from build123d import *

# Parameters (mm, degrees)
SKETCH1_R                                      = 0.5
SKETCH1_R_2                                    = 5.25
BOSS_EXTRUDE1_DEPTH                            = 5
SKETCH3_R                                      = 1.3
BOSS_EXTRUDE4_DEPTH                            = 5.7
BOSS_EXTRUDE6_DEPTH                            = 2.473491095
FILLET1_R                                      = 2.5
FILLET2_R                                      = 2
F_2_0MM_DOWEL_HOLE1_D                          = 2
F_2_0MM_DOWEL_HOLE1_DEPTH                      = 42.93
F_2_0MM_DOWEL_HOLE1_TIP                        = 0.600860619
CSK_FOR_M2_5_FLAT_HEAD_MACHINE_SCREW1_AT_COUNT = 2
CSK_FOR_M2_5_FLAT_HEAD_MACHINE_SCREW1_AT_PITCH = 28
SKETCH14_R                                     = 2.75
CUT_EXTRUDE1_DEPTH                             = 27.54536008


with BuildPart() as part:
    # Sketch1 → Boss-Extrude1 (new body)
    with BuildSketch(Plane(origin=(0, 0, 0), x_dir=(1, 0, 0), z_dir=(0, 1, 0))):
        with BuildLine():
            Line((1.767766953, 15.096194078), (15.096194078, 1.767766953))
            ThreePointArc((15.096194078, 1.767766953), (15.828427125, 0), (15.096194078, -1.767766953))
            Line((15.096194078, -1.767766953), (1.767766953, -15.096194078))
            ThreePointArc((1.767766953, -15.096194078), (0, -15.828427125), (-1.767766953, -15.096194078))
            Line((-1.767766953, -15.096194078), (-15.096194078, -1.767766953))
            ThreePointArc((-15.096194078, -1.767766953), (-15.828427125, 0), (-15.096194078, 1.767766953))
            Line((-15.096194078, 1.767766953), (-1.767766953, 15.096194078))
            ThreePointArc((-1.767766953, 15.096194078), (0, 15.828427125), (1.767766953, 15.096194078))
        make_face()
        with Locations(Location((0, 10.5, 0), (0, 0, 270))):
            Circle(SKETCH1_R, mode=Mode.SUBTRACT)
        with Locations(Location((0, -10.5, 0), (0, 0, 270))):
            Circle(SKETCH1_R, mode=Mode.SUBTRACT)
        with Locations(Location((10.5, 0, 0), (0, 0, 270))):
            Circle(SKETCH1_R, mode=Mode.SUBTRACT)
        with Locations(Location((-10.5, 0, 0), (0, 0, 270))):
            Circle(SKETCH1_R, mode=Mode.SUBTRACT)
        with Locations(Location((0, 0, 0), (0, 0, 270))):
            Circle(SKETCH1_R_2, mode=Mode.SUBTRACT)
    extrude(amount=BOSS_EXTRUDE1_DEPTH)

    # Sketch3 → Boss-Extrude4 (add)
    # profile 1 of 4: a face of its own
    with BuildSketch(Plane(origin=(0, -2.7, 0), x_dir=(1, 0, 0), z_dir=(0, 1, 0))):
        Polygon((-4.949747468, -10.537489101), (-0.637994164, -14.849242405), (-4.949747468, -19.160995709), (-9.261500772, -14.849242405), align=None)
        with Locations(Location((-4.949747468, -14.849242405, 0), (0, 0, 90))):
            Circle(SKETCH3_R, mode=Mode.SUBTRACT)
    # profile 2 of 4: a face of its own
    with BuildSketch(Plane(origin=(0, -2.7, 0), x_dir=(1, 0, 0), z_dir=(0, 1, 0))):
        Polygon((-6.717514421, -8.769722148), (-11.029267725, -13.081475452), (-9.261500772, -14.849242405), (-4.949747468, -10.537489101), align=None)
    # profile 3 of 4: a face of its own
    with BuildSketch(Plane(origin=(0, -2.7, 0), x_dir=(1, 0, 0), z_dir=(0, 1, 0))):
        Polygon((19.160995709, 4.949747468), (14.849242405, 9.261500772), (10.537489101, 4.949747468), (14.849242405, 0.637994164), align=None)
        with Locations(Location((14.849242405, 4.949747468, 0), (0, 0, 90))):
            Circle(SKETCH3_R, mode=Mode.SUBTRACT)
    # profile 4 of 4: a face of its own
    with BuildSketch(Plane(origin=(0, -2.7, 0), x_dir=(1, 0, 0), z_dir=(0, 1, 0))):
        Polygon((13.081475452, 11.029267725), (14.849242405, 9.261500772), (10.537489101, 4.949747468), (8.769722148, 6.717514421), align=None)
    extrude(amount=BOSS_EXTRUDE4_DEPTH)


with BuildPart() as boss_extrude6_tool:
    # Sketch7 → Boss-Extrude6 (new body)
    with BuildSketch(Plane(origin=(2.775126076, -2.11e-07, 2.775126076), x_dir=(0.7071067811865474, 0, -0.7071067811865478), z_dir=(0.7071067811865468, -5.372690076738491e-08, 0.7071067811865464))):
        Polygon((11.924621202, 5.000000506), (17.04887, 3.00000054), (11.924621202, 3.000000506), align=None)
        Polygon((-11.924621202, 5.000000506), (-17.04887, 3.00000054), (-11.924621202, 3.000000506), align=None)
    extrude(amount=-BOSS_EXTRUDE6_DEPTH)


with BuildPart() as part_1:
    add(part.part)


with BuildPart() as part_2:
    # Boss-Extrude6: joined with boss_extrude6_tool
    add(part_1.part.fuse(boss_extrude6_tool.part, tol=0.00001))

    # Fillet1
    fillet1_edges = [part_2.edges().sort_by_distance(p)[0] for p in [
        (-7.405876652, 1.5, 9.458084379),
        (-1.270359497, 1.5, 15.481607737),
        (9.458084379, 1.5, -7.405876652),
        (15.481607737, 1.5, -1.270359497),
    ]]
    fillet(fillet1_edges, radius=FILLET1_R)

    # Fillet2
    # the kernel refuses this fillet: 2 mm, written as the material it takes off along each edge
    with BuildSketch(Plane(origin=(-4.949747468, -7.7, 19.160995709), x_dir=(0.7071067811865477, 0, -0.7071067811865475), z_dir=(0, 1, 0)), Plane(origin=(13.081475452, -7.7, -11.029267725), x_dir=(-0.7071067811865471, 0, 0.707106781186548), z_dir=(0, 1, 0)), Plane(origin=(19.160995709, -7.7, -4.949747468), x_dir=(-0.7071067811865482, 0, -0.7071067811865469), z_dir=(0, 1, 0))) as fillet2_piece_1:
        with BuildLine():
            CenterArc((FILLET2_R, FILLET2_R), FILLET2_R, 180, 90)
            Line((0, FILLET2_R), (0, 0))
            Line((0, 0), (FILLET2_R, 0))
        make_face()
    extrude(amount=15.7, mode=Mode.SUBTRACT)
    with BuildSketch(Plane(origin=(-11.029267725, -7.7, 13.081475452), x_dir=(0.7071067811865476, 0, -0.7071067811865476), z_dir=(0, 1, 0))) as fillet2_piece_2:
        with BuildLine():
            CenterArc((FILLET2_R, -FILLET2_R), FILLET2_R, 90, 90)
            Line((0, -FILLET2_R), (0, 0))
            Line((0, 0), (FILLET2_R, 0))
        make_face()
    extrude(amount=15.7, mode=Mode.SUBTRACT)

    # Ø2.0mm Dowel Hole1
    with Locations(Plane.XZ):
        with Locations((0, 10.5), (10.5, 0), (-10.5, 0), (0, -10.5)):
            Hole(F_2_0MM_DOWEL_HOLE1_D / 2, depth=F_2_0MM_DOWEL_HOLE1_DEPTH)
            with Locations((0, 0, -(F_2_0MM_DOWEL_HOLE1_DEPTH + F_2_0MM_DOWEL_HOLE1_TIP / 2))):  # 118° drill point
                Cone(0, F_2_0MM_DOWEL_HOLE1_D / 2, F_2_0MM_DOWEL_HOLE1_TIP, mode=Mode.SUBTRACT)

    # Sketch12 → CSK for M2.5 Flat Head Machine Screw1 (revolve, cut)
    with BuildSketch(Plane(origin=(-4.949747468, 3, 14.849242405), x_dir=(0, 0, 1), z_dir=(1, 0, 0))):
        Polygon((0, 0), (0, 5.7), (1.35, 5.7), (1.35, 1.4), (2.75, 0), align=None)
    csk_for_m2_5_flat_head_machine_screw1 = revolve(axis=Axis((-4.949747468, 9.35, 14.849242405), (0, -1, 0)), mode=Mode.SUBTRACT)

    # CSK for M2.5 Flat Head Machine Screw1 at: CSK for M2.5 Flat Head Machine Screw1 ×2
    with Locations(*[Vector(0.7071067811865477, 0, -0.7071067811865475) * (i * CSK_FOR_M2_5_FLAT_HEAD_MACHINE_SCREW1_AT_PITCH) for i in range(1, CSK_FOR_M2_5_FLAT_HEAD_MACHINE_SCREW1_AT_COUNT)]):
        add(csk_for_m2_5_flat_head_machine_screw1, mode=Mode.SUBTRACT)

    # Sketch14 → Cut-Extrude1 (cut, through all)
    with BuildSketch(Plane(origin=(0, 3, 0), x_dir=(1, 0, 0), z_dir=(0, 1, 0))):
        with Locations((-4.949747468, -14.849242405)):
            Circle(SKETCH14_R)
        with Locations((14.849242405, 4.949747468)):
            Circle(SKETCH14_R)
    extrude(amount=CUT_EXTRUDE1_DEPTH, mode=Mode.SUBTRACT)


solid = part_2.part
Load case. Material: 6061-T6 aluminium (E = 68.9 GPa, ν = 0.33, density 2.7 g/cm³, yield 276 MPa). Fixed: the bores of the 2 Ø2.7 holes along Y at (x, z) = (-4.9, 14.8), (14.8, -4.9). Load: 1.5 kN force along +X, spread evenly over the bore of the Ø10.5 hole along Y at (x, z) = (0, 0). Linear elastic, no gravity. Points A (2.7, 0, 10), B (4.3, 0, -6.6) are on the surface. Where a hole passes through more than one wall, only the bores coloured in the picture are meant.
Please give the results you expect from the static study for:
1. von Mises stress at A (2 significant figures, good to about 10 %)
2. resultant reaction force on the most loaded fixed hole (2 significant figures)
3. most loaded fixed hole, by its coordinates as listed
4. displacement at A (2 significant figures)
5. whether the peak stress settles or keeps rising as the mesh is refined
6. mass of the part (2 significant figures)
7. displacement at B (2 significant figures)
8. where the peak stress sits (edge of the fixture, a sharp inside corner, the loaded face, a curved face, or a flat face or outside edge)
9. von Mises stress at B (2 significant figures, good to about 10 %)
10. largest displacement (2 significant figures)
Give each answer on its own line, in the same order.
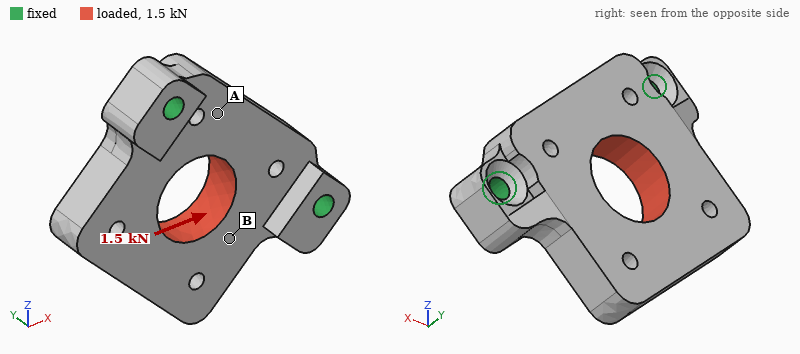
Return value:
18 MPa
980 N
(14.8, -4.9)
6.0 µm
keeps rising
7.5 g
11 µm
edge of the fixture
42 MPa
23 µm
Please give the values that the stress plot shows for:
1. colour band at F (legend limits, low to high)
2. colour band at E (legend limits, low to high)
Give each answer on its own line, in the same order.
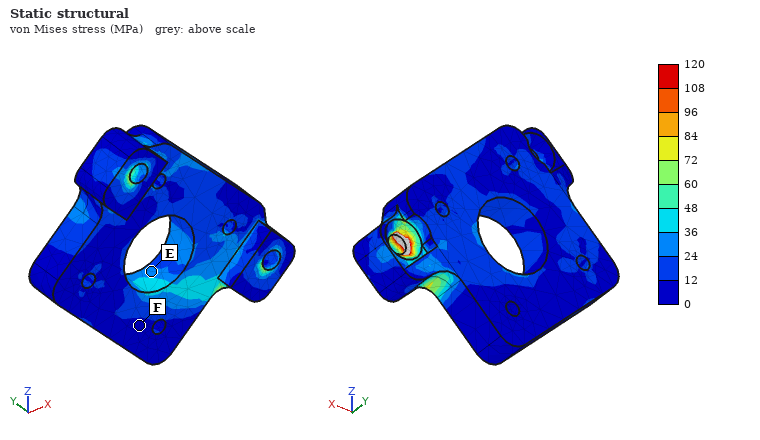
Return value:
0 to 12 MPa
24 to 36 MPa
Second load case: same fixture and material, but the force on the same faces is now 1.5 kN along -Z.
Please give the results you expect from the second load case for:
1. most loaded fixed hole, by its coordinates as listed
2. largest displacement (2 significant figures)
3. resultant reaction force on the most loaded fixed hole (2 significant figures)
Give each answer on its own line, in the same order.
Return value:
(-4.9, 14.8)
23 µm
980 N
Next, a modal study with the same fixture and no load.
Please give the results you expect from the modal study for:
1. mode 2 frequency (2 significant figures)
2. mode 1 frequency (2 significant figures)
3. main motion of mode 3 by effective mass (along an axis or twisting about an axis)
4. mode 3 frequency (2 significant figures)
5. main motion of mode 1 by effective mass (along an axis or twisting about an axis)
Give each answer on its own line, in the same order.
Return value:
18 kHz
7600 Hz
along Y
26 kHz
along Y
